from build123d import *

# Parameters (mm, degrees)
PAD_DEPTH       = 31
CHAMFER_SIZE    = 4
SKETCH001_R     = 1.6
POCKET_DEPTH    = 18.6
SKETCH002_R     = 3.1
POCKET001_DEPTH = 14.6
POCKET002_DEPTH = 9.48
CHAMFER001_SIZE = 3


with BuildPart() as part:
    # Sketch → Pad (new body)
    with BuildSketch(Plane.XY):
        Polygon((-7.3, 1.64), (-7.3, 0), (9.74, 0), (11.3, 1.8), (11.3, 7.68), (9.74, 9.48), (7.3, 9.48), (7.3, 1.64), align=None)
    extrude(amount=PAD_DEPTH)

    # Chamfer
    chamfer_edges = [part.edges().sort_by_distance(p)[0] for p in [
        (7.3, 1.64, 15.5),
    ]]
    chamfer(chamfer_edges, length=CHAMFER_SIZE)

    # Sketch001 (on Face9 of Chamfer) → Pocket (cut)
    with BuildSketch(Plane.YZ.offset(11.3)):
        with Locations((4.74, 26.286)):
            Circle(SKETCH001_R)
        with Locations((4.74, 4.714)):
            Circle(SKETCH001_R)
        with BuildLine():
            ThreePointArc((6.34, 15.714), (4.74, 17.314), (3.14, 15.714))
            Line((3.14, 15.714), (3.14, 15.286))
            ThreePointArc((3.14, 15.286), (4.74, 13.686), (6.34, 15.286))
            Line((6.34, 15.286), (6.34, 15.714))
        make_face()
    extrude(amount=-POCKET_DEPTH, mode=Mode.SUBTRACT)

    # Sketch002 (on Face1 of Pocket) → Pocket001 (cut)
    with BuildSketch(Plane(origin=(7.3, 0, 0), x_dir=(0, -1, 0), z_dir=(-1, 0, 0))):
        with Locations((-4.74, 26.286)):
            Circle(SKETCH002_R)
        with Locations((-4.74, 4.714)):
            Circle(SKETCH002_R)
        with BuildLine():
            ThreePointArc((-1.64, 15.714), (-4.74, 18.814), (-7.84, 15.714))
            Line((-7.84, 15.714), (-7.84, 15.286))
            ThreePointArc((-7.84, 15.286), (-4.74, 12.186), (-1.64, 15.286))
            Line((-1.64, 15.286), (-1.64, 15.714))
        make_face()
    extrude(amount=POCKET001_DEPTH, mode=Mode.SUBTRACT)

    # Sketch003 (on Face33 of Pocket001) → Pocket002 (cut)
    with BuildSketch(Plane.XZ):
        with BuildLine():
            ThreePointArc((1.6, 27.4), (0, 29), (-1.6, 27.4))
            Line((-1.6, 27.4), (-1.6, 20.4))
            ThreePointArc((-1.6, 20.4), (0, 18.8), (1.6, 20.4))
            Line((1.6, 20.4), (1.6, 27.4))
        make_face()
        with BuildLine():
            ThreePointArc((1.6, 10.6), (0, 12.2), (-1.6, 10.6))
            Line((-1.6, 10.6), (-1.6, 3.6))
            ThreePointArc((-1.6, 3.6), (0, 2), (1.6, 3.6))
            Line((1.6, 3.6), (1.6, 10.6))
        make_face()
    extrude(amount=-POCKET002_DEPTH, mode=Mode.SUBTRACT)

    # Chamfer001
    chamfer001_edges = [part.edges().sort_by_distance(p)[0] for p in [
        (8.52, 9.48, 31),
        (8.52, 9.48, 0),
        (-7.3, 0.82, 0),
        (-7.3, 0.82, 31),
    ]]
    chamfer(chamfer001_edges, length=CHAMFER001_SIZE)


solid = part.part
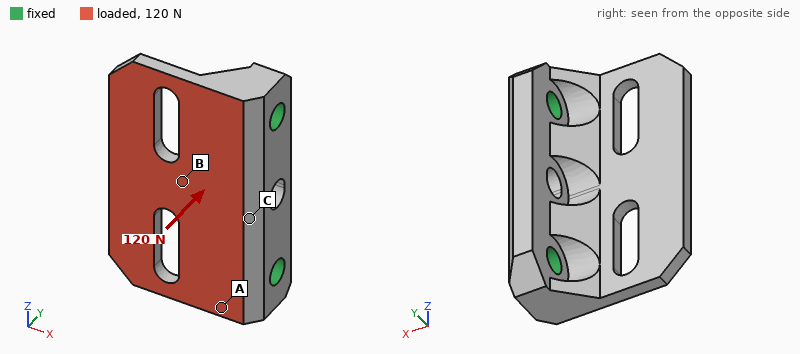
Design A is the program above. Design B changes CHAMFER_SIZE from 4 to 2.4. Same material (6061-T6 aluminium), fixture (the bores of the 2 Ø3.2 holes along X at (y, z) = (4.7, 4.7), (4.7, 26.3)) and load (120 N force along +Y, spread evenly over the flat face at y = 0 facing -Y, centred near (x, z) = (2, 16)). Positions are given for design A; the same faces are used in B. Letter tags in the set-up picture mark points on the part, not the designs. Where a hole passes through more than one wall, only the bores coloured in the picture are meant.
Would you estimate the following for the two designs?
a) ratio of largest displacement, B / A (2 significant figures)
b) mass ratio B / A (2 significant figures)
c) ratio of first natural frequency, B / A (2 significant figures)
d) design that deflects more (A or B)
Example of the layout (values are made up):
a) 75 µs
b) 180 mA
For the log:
a) 1.3
b) 0.95
c) 0.89
d) B
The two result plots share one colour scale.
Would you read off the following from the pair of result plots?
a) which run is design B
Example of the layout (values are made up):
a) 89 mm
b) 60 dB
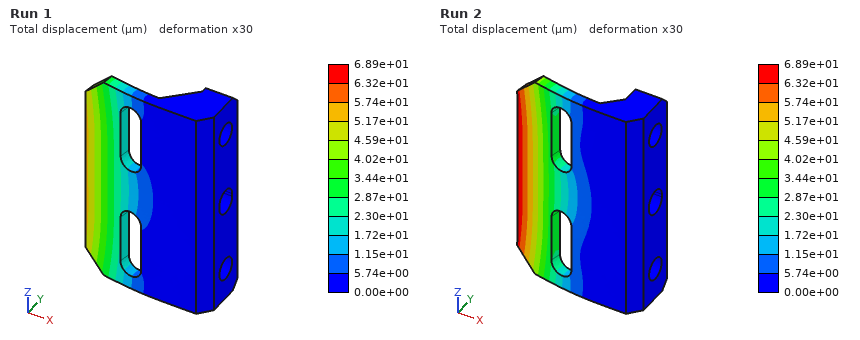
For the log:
a) Run 2
